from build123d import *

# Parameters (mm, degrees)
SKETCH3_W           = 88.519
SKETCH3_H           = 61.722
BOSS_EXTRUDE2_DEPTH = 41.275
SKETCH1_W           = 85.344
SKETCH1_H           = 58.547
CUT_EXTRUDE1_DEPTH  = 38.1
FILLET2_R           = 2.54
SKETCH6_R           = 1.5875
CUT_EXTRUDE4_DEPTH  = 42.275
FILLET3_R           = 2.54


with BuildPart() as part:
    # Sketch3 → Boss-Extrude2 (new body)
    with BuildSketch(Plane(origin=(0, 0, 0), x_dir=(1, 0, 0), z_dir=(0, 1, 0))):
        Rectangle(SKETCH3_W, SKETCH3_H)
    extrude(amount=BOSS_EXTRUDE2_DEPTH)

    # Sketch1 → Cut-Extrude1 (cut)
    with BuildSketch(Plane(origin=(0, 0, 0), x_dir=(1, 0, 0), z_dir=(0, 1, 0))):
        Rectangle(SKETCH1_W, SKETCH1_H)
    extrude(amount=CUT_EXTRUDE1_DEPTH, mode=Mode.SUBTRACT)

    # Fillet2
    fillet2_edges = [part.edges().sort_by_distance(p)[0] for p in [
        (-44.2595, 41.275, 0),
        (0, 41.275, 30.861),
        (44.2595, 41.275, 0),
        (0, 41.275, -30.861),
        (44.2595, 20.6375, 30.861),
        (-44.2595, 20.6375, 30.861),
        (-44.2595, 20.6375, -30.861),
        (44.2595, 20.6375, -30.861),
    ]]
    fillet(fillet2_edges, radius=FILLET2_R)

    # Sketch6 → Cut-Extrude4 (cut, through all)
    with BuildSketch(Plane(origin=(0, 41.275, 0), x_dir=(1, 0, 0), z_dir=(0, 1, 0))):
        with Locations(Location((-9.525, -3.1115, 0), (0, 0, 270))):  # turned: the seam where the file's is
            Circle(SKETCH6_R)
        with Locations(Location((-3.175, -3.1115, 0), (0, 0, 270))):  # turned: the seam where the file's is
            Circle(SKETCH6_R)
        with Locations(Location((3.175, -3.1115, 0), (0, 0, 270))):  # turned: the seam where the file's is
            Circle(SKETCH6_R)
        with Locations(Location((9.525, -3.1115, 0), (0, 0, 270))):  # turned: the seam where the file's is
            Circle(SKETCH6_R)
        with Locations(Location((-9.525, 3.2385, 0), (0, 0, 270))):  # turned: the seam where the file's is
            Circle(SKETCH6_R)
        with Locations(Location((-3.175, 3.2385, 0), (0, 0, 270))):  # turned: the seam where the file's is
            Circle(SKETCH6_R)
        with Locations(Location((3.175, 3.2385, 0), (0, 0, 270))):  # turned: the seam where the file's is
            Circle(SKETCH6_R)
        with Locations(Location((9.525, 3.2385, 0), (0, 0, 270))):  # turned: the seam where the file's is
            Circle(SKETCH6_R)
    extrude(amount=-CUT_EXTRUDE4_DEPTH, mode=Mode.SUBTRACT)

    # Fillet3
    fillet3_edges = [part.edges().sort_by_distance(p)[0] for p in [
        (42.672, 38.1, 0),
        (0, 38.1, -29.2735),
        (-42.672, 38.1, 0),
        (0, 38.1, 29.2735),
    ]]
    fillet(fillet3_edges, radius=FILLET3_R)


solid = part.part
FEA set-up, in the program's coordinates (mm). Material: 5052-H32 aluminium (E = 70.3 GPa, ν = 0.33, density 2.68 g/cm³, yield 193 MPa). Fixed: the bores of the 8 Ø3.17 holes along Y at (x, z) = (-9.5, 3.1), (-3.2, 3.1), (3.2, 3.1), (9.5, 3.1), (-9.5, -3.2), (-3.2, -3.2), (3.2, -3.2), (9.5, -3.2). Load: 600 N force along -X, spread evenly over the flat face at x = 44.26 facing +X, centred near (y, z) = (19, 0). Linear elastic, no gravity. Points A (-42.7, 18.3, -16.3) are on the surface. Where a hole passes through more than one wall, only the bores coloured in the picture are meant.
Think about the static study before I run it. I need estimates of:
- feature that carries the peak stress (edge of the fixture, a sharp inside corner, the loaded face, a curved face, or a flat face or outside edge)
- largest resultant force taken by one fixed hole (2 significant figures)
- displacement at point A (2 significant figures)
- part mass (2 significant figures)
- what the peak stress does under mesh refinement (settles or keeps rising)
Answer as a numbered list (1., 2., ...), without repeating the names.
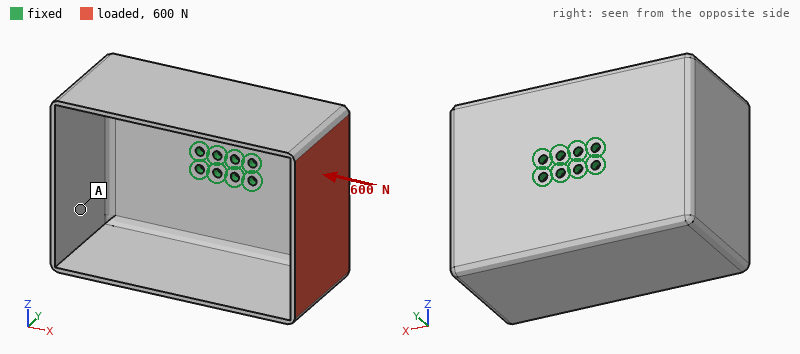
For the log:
1. edge of the fixture
2. 250 N
3. 0.16 mm
4. 93 g
5. keeps rising
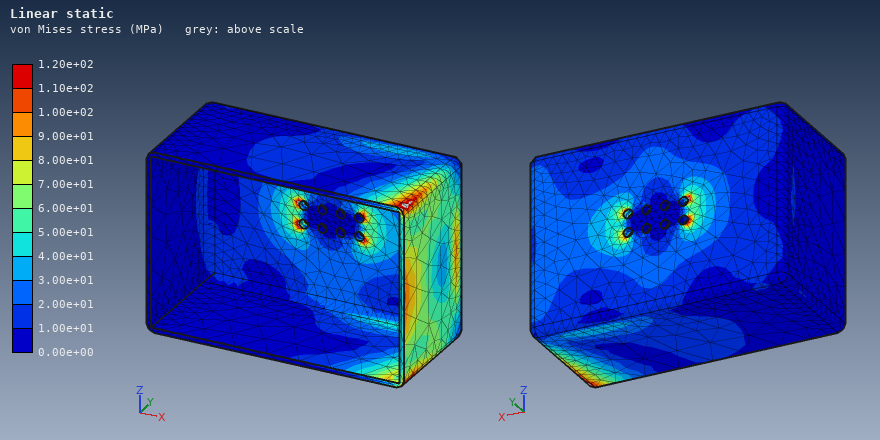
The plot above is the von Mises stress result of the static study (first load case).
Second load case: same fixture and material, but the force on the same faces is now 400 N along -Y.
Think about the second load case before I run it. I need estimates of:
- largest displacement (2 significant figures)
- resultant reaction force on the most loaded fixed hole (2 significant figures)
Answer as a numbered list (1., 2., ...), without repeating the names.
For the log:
1. 0.34 mm
2. 400 N
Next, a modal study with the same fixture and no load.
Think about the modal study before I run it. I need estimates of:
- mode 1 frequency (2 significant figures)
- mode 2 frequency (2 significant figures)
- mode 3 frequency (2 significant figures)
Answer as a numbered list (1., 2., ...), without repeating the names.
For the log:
1. 910 Hz
2. 950 Hz
3. 960 Hz
